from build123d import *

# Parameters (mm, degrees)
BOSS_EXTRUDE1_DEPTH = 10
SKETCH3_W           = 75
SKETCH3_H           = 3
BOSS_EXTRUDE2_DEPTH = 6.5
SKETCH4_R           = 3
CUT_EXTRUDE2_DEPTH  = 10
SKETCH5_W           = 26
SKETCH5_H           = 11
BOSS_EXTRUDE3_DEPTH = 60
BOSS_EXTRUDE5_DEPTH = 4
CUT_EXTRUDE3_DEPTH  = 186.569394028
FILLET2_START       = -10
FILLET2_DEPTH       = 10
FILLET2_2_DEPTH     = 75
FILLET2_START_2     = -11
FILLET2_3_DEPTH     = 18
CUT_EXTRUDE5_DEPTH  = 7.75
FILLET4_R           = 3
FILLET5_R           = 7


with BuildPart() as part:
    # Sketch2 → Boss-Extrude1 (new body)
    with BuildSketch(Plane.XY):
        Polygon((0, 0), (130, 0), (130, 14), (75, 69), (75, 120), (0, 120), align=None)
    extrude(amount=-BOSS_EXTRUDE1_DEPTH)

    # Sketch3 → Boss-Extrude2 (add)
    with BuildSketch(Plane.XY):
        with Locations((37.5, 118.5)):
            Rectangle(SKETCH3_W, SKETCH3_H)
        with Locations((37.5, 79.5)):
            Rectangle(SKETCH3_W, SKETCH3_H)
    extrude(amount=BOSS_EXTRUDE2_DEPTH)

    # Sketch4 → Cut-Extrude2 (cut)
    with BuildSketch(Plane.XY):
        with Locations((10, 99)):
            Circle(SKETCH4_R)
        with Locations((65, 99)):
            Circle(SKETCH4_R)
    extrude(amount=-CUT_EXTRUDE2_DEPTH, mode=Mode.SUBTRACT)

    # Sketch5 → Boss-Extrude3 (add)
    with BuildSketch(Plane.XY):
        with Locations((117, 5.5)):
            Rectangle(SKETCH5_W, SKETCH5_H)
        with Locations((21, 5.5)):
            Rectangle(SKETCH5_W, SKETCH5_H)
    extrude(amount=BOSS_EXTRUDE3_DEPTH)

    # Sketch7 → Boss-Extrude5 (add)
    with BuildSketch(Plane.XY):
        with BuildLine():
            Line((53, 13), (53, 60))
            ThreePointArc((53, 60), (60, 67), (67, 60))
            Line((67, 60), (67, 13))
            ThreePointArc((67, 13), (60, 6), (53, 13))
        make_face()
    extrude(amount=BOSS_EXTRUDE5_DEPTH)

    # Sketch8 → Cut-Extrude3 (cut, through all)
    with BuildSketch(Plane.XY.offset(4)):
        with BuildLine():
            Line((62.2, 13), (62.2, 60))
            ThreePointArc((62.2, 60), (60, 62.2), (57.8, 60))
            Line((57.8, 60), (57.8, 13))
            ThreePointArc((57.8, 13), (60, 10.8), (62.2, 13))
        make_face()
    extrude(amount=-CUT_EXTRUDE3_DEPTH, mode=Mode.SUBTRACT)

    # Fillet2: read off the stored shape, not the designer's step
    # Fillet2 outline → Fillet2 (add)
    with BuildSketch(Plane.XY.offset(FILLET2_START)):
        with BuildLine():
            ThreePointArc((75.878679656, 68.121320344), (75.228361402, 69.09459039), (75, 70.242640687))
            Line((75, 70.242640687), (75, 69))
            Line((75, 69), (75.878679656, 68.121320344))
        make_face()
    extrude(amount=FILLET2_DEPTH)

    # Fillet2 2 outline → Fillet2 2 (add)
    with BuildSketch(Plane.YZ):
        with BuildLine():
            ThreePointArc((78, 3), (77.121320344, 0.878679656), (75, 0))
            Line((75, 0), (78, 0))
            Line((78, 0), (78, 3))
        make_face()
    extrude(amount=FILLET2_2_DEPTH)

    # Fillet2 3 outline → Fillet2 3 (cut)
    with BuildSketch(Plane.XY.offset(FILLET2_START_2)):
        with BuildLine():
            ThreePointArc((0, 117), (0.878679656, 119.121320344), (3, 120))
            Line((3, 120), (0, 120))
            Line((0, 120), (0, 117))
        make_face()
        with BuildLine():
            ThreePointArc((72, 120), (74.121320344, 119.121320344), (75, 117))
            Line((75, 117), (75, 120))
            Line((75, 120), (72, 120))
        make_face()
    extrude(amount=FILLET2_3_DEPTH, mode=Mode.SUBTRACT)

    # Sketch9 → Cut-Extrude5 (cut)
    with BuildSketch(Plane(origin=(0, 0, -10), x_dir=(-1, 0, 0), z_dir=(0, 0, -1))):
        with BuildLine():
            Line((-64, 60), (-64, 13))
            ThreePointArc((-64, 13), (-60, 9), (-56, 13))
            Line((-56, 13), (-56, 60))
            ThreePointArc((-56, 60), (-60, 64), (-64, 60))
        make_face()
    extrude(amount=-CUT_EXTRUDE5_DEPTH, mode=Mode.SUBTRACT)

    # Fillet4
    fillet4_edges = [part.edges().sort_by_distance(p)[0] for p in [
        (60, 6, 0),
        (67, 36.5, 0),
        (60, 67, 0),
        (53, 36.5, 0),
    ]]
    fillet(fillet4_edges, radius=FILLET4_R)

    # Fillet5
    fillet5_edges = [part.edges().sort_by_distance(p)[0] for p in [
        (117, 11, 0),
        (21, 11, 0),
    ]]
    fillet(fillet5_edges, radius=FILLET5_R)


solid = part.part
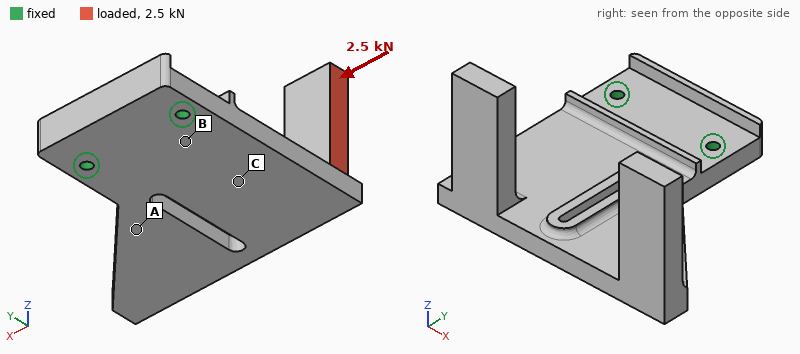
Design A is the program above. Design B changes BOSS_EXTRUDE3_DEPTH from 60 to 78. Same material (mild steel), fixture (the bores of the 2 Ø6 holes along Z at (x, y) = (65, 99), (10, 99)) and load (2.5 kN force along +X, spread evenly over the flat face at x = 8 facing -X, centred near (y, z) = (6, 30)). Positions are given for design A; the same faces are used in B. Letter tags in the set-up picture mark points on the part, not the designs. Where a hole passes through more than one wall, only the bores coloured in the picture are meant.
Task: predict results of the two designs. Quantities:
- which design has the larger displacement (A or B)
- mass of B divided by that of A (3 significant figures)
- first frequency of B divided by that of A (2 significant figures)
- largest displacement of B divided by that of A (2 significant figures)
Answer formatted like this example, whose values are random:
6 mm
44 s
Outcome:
B
1.07
0.88
1.6
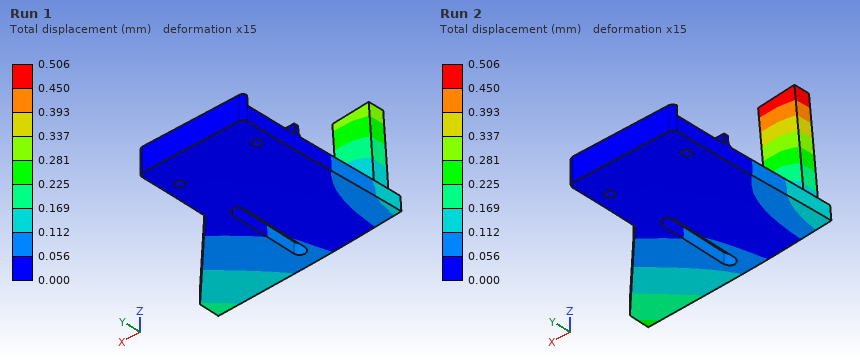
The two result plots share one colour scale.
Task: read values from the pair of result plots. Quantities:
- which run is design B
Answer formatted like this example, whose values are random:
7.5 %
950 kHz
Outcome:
Run 2
